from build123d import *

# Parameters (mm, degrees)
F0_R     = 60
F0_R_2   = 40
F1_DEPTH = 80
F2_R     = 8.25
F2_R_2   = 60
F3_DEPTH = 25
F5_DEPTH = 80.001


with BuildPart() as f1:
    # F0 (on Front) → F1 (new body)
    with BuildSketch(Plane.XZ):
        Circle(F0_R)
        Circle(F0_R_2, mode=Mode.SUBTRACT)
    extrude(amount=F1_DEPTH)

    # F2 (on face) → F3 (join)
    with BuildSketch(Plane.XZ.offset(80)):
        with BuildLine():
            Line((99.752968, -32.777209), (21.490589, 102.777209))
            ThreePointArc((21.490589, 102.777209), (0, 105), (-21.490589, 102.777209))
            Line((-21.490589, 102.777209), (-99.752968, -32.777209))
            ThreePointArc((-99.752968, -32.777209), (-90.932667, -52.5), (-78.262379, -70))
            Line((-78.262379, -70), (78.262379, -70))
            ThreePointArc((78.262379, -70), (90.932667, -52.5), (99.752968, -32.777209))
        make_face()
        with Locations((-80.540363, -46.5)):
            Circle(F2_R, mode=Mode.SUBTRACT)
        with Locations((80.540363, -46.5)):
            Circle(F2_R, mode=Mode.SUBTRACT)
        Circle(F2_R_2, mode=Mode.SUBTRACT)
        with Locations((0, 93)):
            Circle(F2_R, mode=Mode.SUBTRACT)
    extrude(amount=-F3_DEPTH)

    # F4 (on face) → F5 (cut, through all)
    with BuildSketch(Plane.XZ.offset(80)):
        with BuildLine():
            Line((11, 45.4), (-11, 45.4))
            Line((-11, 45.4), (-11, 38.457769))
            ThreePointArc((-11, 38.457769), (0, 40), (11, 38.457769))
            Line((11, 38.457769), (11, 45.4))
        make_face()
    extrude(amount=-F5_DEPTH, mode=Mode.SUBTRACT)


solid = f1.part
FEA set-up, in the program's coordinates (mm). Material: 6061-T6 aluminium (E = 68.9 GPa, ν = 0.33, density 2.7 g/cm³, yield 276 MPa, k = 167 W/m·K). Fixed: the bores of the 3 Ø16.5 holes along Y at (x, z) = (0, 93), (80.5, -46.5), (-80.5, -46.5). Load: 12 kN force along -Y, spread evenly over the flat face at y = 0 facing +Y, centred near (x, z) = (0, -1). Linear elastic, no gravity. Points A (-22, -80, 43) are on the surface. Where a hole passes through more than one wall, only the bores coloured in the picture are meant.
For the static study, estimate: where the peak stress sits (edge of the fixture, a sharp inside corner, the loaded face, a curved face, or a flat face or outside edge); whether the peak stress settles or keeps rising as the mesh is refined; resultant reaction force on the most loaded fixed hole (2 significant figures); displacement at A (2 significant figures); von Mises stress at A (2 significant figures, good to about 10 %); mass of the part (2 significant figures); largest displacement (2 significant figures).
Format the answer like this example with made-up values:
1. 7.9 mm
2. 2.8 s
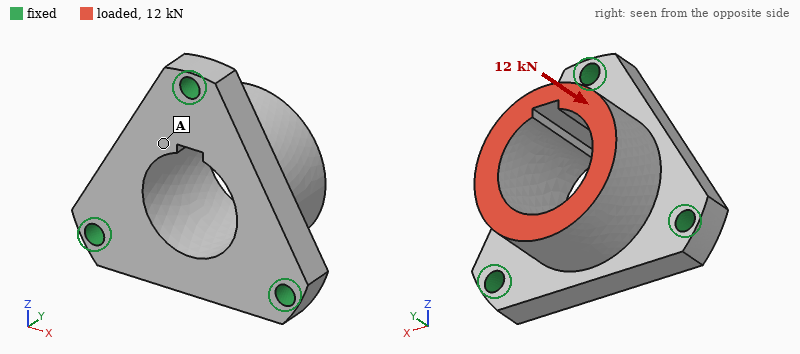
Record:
1. edge of the fixture
2. keeps rising
3. 4.3 kN
4. 12 µm
5. 4.1 MPa
6. 2.1 kg
7. 14 µm
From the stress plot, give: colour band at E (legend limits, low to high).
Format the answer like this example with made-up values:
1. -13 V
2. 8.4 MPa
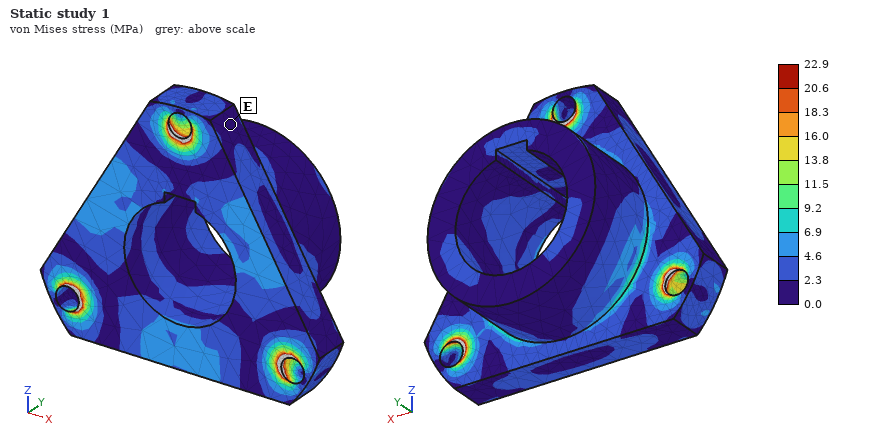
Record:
1. 0.0 to 2.3 MPa
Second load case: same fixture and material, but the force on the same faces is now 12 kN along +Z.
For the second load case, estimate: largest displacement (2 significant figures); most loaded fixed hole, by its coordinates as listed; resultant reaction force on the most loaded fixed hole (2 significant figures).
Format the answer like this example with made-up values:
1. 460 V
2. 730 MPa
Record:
1. 51 µm
2. (0, 93)
3. 7.9 kN
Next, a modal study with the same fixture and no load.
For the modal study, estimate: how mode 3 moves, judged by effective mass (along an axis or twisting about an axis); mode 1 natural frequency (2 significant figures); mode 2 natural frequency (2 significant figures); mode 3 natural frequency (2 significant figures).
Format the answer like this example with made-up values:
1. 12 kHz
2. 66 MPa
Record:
1. along Y
2. 3600 Hz
3. 3700 Hz
4. 3900 Hz
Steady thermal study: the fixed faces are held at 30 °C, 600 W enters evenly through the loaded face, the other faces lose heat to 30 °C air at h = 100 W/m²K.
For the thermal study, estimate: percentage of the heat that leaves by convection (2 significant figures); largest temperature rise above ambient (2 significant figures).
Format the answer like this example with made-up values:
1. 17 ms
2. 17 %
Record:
1. 34 %
2. 52 K
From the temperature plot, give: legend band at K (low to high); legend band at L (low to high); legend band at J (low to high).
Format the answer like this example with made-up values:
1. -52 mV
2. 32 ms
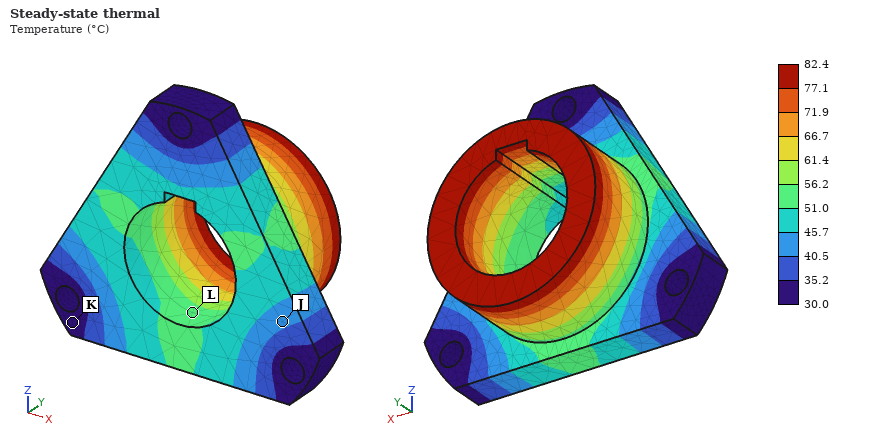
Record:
1. 30.0 to 35.2 °C
2. 51.0 to 56.2 °C
3. 40.5 to 45.7 °C
